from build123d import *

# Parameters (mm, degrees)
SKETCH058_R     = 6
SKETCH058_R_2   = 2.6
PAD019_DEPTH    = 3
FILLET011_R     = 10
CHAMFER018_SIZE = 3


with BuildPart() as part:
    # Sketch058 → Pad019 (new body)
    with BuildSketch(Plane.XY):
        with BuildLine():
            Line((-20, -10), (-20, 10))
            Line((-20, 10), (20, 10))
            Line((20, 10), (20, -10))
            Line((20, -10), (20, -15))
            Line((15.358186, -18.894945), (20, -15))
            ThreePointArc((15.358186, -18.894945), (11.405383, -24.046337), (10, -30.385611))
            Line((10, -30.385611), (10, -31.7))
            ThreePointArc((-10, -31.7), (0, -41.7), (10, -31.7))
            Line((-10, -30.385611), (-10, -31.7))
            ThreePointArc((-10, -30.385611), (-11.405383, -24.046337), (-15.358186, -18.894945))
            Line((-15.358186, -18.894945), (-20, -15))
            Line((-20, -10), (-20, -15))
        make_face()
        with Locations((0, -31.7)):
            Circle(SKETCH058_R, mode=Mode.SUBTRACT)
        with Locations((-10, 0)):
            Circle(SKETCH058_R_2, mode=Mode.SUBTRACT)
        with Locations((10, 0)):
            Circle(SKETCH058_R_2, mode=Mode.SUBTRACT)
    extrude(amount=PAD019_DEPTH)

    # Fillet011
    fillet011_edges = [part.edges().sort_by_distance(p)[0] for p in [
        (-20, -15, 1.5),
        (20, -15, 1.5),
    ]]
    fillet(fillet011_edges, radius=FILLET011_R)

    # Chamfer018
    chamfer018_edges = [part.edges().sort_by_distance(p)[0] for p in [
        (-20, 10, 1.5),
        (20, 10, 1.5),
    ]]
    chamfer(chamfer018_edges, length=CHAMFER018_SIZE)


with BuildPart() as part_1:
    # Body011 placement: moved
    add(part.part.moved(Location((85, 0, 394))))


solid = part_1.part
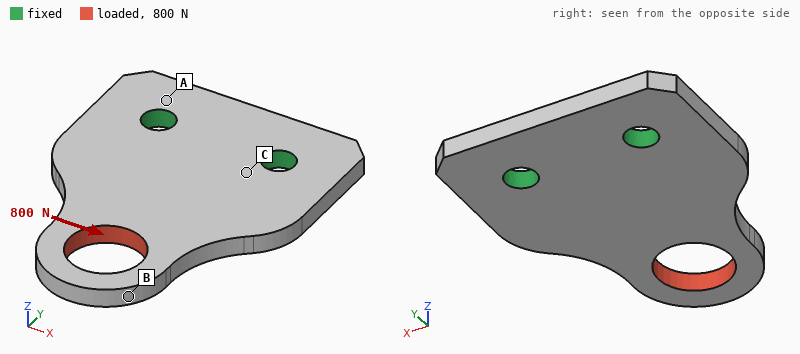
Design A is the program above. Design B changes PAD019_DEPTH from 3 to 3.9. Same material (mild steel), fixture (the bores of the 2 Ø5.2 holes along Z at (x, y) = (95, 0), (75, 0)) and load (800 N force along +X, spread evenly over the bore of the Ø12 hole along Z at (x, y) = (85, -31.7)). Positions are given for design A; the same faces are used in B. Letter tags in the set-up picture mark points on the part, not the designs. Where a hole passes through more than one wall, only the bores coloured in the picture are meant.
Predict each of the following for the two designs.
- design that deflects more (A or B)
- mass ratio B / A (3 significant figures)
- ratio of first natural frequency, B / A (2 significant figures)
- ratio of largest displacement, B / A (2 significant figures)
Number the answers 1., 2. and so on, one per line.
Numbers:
1. A
2. 1.30
3. 1.3
4. 0.77
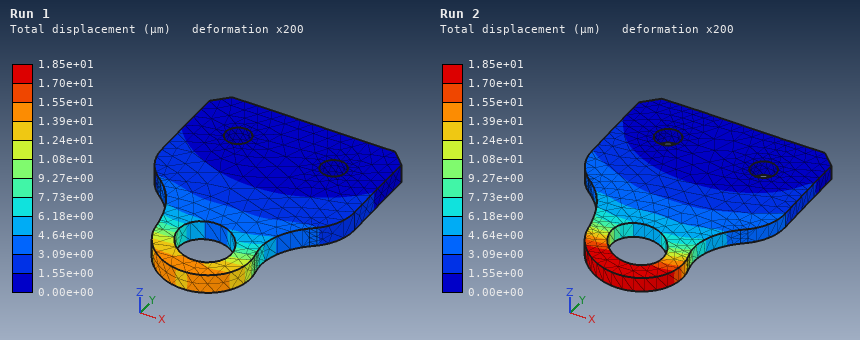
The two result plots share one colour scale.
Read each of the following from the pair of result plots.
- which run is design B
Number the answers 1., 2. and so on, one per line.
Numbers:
1. Run 1
